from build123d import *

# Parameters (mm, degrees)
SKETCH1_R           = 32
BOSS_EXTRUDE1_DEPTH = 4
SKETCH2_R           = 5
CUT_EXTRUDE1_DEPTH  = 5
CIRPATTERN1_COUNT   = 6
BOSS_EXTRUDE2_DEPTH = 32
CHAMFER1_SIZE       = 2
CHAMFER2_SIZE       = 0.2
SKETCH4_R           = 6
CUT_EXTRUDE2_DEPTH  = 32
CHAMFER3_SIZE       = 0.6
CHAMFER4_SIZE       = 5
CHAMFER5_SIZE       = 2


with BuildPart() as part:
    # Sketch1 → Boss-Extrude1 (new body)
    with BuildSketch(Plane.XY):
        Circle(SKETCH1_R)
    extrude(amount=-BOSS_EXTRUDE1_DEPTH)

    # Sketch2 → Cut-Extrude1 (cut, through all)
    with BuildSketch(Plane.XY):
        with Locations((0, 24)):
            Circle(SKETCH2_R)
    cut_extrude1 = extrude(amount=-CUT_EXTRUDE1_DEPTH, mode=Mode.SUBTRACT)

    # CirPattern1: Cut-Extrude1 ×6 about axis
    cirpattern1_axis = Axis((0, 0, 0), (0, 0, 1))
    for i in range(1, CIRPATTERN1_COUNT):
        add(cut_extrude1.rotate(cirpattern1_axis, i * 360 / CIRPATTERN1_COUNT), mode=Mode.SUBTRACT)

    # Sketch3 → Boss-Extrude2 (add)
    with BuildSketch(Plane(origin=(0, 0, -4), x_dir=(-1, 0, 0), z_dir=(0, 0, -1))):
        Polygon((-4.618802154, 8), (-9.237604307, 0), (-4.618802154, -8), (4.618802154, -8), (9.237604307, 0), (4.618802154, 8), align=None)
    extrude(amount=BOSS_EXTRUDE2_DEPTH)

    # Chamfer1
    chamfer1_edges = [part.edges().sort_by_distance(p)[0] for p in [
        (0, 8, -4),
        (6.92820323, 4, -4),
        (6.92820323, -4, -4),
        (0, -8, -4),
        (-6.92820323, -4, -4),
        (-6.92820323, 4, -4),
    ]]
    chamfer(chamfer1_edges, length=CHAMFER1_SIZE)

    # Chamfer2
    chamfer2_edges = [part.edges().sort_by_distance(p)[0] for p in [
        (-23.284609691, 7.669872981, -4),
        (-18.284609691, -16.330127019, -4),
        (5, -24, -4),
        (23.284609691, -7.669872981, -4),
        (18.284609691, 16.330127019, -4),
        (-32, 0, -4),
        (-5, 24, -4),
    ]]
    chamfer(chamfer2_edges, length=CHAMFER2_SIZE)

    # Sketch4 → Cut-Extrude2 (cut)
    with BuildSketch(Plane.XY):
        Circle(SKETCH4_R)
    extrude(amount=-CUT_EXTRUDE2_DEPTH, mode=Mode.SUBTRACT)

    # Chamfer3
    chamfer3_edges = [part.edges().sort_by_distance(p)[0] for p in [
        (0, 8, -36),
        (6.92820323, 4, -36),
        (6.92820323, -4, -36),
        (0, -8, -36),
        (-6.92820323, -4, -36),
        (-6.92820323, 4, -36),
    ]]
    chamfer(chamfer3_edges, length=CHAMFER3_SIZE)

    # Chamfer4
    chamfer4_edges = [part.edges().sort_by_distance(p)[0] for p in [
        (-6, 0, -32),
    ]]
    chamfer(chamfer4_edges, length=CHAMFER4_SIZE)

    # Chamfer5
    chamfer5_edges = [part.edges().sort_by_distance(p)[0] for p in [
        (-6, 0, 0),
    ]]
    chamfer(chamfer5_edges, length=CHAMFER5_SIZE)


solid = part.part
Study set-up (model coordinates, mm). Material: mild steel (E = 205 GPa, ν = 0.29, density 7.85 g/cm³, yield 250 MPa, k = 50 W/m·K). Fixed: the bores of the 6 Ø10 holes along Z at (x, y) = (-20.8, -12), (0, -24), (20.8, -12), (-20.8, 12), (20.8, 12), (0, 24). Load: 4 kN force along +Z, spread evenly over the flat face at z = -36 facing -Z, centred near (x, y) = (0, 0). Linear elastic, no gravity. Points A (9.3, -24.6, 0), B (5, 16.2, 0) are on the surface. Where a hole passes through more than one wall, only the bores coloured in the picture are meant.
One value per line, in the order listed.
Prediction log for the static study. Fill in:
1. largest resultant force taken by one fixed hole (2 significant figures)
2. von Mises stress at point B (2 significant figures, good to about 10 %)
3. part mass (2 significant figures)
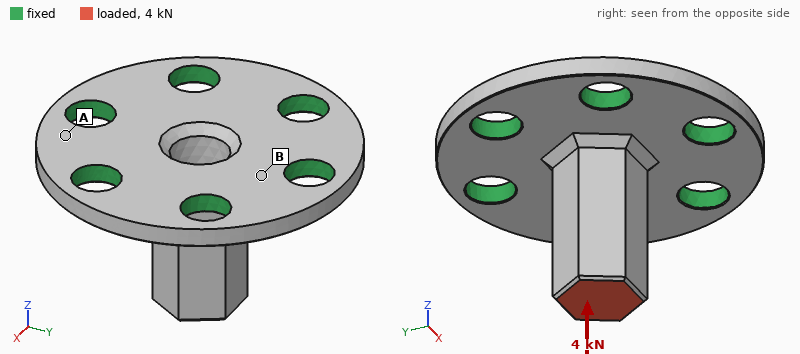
850 N
48 MPa
120 g
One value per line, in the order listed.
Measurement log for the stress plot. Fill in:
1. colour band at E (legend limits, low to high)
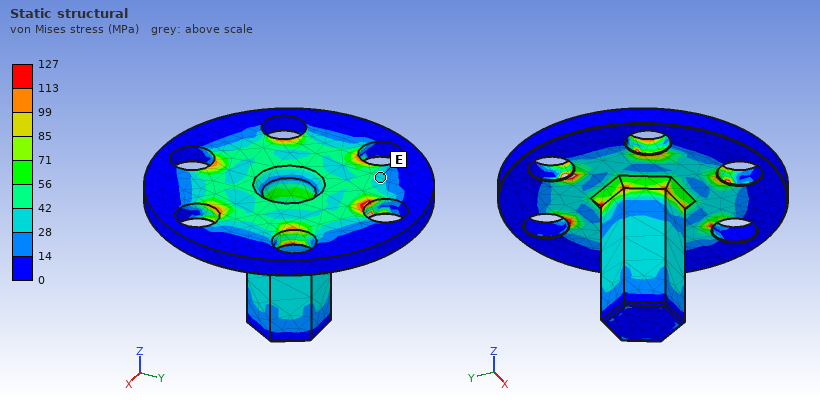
28 to 42 MPa
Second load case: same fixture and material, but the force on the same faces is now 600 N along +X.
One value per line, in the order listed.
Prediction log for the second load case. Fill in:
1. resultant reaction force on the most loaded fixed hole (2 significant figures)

420 N
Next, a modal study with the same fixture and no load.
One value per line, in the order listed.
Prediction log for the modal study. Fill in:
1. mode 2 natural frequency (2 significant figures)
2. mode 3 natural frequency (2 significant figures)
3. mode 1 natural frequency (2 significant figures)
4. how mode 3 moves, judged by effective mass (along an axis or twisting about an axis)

6000 Hz
14 kHz
6000 Hz
along Z
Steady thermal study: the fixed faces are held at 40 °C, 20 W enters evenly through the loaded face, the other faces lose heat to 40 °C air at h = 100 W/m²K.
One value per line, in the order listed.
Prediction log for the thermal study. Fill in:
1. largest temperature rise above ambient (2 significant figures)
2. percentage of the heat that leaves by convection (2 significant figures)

76 K
57 %
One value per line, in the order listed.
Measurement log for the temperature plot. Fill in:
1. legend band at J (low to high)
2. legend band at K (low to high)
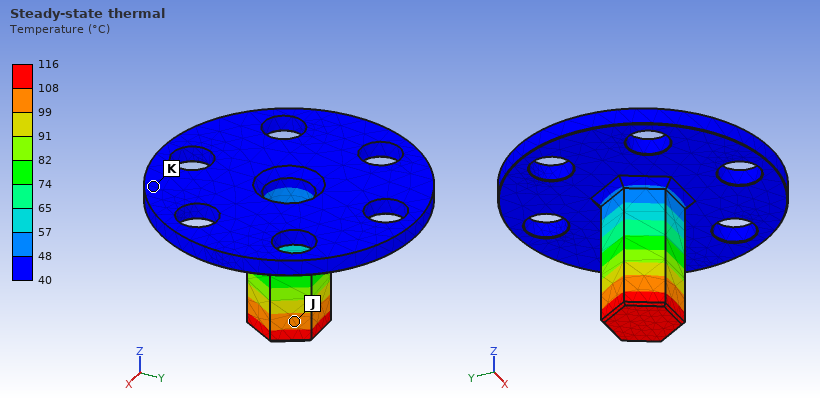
99 to 108 °C
40 to 48 °C
